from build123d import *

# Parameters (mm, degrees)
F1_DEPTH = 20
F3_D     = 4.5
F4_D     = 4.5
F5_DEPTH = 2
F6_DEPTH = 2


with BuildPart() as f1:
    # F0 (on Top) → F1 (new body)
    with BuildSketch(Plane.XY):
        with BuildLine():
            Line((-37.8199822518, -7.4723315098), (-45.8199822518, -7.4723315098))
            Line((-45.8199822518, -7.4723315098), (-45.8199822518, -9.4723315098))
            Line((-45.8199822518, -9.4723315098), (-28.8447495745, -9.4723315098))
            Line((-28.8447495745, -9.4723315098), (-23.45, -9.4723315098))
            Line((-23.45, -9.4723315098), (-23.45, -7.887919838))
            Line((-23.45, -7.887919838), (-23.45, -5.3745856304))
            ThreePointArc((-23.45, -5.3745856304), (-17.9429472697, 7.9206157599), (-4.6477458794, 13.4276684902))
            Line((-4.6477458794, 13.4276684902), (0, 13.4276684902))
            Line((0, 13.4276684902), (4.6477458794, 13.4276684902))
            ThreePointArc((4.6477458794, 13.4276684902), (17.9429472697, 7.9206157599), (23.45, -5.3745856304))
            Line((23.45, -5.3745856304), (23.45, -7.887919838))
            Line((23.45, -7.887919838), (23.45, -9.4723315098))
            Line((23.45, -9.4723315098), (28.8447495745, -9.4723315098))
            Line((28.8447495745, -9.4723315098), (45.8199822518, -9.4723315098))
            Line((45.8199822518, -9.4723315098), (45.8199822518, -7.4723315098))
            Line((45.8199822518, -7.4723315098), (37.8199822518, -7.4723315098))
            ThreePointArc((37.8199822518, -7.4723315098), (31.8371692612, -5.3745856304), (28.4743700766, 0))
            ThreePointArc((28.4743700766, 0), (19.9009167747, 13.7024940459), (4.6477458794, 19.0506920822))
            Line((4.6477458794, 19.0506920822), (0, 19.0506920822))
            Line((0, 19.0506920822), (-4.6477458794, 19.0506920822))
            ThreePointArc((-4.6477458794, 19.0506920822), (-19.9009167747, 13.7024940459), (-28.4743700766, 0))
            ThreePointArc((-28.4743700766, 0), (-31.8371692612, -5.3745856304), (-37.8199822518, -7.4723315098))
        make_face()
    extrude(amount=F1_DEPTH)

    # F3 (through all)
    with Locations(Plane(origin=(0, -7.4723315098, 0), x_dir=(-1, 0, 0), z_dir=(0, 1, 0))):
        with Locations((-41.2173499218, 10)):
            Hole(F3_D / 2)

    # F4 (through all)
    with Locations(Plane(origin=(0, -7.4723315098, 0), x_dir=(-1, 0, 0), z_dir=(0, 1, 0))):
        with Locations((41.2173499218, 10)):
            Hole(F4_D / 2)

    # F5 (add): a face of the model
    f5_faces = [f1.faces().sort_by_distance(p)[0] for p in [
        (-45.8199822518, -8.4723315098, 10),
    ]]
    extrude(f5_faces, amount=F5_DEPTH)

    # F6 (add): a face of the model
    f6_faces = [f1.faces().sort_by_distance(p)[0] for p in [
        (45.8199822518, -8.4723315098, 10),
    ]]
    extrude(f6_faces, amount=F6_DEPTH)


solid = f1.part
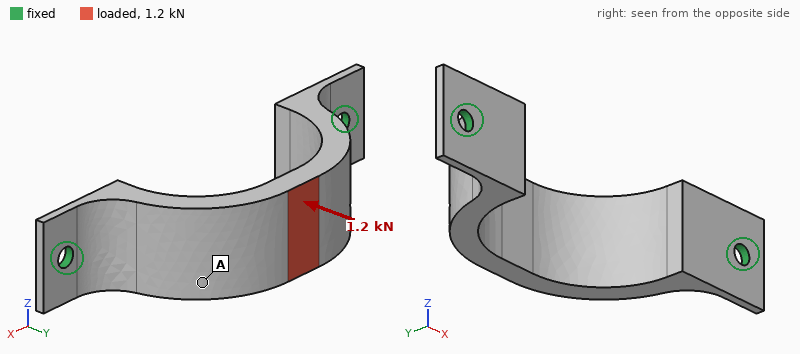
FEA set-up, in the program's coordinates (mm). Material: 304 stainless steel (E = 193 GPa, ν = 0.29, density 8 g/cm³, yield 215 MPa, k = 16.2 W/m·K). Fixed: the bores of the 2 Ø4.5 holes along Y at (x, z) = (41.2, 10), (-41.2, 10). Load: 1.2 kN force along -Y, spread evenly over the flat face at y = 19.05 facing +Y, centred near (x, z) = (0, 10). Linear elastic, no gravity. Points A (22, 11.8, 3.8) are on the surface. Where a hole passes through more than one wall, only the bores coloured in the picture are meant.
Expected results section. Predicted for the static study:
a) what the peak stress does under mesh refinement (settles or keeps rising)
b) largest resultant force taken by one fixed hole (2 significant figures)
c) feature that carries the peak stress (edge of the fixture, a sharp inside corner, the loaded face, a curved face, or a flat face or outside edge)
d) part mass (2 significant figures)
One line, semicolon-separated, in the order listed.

keeps rising; 910 N; edge of the fixture; 93 g
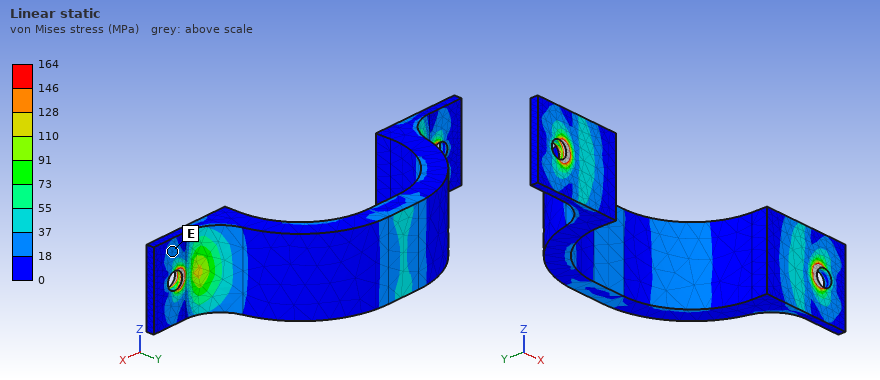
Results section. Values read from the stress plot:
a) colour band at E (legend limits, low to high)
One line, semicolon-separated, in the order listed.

18 to 37 MPa
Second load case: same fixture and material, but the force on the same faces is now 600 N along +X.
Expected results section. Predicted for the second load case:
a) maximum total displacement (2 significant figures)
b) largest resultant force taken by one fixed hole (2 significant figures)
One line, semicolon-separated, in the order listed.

7.8 µm; 370 N
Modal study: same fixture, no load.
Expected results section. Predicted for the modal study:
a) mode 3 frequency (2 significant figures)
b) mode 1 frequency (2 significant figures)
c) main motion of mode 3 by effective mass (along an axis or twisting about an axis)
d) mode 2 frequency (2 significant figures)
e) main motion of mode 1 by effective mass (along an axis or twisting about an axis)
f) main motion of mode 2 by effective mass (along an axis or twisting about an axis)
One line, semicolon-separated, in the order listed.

4900 Hz; 1300 Hz; along Y; 4600 Hz; along Z; along X
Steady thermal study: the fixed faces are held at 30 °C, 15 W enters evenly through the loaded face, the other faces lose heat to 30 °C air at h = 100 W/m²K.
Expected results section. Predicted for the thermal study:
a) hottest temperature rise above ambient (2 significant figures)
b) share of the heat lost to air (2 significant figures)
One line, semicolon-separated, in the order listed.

86 K; 93 %
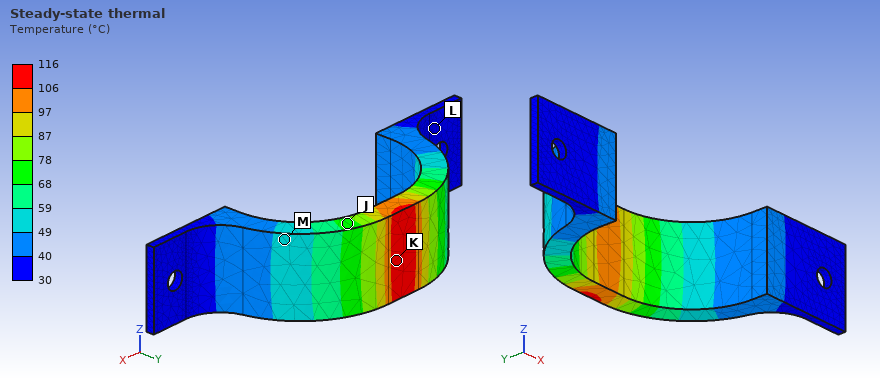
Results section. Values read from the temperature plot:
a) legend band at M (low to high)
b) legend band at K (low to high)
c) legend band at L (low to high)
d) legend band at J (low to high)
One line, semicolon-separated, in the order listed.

49 to 59 °C; 106 to 116 °C; 30 to 40 °C; 68 to 78 °C
